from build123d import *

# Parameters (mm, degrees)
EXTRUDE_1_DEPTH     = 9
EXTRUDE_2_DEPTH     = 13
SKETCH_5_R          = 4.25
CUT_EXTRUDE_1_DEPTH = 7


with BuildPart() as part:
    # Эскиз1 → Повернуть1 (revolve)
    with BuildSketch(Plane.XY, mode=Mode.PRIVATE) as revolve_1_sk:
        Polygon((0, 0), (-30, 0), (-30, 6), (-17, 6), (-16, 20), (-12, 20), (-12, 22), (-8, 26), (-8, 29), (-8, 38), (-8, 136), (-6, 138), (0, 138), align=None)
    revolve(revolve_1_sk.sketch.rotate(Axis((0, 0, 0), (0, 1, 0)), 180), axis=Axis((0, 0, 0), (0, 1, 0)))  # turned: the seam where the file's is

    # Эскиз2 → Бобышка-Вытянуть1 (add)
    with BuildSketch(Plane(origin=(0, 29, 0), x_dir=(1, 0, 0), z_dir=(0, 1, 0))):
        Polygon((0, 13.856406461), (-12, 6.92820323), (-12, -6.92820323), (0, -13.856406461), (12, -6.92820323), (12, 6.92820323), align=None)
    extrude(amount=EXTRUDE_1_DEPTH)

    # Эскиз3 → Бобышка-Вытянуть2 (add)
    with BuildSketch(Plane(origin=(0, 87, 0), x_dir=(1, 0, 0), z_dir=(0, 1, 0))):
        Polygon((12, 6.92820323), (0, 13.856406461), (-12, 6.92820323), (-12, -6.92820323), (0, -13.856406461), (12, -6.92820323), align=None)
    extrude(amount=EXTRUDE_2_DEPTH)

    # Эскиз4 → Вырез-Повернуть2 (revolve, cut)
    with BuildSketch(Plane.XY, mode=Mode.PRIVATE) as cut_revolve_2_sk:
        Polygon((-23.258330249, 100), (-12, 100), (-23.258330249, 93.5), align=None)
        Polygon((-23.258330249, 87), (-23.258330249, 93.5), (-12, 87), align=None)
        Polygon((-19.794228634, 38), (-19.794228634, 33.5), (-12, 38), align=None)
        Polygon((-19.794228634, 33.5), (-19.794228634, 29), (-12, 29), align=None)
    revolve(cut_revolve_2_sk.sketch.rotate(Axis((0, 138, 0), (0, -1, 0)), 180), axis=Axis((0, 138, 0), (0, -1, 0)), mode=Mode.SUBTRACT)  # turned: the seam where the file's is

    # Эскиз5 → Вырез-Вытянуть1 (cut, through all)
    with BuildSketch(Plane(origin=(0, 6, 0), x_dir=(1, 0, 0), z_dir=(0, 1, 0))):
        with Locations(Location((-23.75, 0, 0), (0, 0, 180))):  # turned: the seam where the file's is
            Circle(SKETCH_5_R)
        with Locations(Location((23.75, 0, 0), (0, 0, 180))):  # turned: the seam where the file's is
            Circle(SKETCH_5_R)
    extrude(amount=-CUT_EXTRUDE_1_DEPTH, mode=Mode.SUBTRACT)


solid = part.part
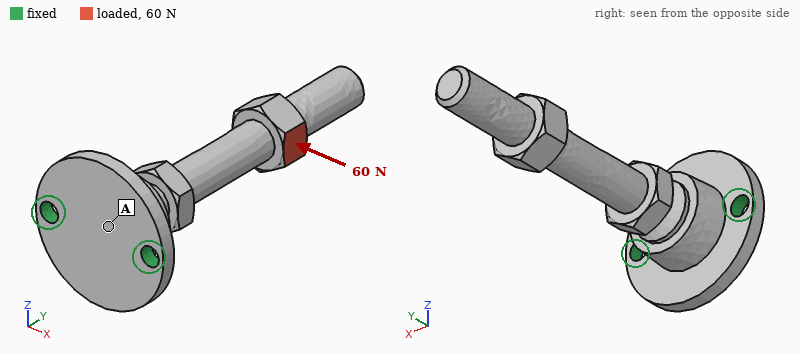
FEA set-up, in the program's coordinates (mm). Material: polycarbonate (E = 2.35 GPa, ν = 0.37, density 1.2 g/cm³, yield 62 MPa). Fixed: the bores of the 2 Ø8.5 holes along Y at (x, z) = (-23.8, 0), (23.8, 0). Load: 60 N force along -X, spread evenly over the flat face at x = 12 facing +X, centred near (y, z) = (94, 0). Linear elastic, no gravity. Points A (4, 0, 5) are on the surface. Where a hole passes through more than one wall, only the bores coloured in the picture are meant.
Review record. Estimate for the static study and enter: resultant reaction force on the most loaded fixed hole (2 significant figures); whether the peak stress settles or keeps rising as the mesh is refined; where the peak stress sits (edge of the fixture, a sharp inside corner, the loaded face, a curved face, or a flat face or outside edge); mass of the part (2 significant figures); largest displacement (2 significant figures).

150 N
keeps rising
a sharp inside corner
71 g
1.8 mm
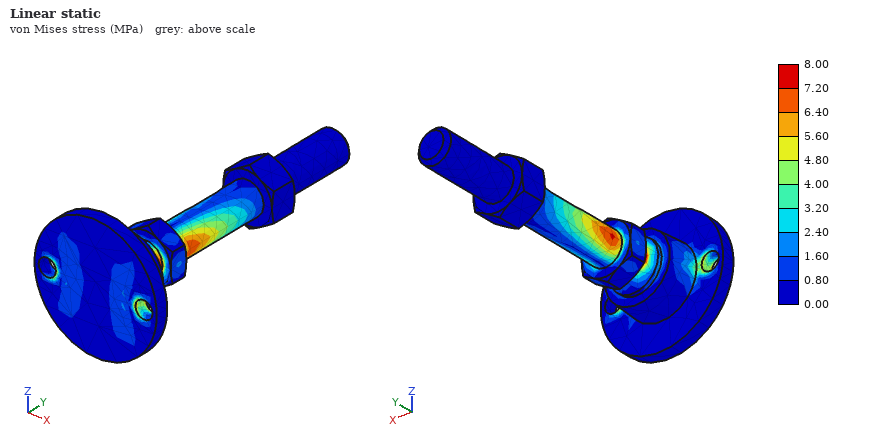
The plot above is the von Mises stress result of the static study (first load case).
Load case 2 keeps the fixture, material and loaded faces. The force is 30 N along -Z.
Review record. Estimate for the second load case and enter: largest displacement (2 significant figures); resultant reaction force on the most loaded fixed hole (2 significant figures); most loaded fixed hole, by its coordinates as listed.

1.5 mm
22 N
(23.8, 0)
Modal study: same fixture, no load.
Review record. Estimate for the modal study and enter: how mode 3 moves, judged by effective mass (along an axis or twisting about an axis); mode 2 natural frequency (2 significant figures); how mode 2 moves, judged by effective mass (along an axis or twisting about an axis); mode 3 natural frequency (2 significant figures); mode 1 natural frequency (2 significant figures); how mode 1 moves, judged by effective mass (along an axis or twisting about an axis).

along Z
220 Hz
along X
900 Hz
170 Hz
along Z
